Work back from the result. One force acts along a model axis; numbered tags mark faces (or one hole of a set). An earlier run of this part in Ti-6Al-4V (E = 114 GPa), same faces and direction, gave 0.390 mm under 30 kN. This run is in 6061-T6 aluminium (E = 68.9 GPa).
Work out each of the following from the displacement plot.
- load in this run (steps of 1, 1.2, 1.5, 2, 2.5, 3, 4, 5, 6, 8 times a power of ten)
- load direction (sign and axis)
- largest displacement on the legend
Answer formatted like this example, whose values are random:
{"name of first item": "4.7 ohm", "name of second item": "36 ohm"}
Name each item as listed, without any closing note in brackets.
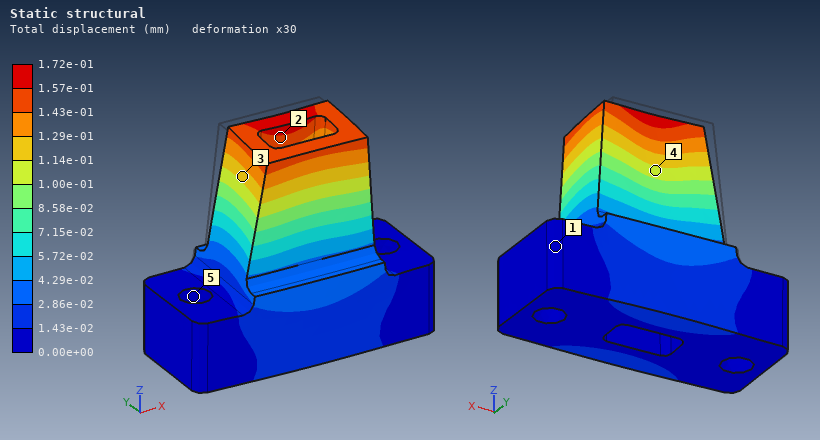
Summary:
{"load in this run": "8 kN", "load direction": "-Y", "largest displacement on the legend": "1.72e-01 mm"}
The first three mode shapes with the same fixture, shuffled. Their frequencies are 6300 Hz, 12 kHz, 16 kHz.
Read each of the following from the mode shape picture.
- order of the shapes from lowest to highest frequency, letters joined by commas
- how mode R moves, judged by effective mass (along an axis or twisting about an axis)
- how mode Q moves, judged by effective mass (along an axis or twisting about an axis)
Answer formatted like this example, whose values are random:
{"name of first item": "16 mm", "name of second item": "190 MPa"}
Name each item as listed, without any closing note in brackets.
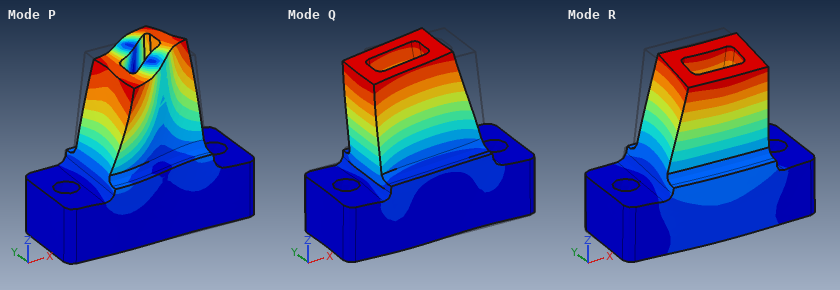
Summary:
{"order of the shapes from lowest to highest frequency, letters joined by commas": "R, Q, P", "how mode R moves, judged by effective mass": "along Y", "how mode Q moves, judged by effective mass": "along X"}
